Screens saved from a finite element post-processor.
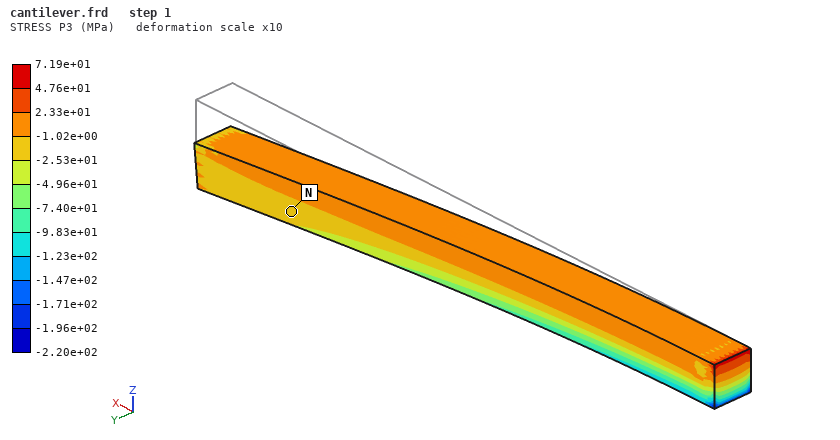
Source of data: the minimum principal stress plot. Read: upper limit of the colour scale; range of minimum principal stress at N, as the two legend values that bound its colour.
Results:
7.19e+01 MPa
-2.53e+01 to -1.02e+00 MPa
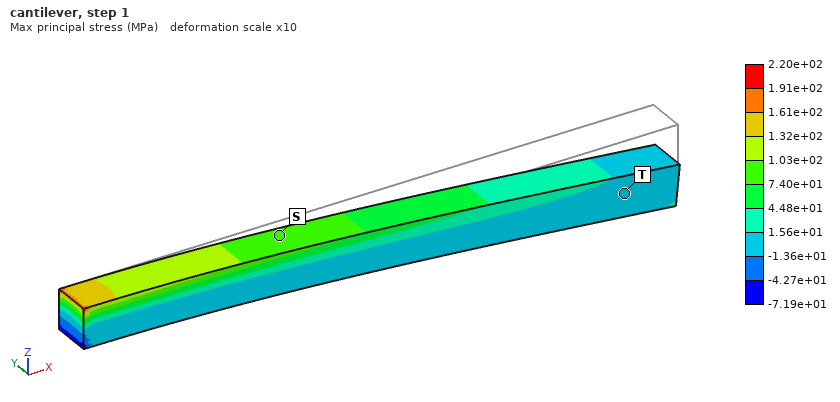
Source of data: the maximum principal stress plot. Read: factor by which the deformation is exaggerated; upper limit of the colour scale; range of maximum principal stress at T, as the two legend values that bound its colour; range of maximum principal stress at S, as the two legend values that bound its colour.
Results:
10
2.20e+02 MPa
-1.36e+01 to 1.56e+01 MPa
7.40e+01 to 1.03e+02 MPa
